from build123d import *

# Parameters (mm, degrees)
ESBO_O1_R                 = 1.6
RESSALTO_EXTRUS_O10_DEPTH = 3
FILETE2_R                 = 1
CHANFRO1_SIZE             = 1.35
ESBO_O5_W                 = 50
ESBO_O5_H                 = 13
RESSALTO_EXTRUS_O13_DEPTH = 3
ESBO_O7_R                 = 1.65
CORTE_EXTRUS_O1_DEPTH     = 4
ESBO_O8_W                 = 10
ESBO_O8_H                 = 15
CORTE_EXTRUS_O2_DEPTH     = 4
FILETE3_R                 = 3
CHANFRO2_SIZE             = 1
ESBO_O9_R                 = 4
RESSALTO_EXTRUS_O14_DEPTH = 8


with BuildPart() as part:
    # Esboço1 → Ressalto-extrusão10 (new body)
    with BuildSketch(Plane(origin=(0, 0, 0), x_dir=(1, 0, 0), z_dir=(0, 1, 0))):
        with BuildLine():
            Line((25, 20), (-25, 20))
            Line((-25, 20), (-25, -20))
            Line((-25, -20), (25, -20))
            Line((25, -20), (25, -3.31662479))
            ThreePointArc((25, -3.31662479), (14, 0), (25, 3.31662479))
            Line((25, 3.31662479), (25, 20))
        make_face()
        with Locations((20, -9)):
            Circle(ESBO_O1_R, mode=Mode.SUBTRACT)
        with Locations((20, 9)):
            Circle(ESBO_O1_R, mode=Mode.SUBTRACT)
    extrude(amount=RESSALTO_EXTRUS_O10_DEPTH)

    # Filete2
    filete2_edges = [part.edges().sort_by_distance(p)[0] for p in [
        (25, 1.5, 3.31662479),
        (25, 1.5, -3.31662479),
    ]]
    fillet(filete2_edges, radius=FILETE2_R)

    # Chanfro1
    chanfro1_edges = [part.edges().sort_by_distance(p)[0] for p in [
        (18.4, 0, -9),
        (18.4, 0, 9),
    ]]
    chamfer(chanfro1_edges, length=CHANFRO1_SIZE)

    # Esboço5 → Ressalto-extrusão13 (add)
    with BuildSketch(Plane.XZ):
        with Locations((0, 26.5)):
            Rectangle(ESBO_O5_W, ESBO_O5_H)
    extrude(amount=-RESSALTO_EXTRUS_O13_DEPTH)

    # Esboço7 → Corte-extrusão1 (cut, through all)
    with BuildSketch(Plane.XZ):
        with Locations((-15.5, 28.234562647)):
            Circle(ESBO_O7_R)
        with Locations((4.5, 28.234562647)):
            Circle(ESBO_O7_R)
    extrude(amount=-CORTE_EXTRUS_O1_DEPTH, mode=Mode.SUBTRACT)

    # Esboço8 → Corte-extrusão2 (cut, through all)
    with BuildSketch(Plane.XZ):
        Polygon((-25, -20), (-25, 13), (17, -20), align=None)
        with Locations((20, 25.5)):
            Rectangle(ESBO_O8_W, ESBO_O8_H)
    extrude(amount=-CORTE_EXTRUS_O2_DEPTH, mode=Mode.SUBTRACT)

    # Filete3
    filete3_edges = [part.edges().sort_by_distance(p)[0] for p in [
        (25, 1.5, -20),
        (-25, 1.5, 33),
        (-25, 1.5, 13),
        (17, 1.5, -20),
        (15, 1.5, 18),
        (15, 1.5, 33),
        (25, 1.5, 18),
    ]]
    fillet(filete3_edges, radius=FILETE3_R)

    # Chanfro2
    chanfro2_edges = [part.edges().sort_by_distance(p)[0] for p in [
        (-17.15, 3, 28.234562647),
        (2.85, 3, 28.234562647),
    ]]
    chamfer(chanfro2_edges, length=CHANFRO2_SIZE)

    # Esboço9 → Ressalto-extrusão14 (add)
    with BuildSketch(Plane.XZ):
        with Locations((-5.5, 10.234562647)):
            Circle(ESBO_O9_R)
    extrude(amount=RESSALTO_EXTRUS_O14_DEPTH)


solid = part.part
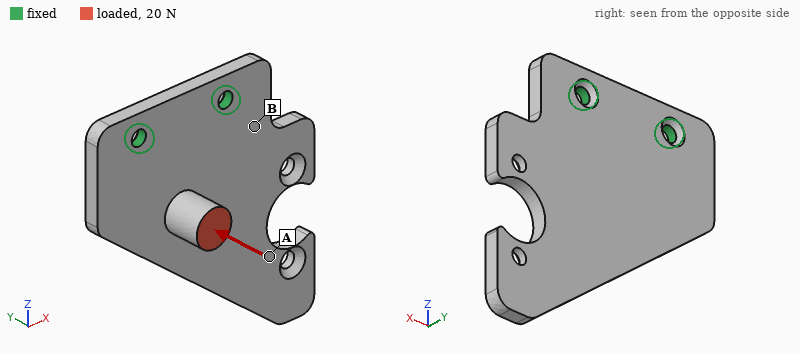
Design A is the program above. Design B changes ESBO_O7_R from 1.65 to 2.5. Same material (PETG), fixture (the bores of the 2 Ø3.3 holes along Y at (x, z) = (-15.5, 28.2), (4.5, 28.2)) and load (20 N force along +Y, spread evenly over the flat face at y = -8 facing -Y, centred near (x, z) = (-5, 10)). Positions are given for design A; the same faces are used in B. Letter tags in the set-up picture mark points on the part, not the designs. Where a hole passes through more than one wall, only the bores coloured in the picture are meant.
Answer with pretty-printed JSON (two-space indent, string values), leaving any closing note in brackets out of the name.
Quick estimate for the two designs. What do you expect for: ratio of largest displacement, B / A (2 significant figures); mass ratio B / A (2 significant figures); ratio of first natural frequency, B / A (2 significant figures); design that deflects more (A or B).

{
  "ratio of largest displacement, B / A": "0.81",
  "mass ratio B / A": "0.99",
  "ratio of first natural frequency, B / A": "1.1",
  "design that deflects more": "A"
}
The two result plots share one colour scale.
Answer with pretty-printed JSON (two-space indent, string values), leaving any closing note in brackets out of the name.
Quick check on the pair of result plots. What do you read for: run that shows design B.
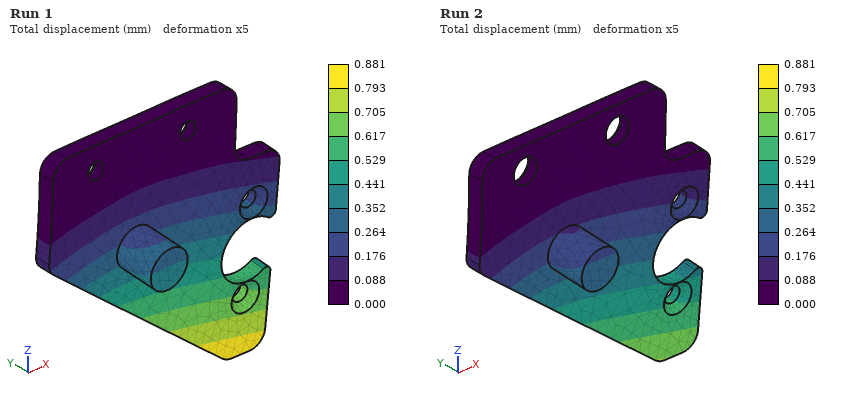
{
  "run that shows design B": "Run 2"
}
